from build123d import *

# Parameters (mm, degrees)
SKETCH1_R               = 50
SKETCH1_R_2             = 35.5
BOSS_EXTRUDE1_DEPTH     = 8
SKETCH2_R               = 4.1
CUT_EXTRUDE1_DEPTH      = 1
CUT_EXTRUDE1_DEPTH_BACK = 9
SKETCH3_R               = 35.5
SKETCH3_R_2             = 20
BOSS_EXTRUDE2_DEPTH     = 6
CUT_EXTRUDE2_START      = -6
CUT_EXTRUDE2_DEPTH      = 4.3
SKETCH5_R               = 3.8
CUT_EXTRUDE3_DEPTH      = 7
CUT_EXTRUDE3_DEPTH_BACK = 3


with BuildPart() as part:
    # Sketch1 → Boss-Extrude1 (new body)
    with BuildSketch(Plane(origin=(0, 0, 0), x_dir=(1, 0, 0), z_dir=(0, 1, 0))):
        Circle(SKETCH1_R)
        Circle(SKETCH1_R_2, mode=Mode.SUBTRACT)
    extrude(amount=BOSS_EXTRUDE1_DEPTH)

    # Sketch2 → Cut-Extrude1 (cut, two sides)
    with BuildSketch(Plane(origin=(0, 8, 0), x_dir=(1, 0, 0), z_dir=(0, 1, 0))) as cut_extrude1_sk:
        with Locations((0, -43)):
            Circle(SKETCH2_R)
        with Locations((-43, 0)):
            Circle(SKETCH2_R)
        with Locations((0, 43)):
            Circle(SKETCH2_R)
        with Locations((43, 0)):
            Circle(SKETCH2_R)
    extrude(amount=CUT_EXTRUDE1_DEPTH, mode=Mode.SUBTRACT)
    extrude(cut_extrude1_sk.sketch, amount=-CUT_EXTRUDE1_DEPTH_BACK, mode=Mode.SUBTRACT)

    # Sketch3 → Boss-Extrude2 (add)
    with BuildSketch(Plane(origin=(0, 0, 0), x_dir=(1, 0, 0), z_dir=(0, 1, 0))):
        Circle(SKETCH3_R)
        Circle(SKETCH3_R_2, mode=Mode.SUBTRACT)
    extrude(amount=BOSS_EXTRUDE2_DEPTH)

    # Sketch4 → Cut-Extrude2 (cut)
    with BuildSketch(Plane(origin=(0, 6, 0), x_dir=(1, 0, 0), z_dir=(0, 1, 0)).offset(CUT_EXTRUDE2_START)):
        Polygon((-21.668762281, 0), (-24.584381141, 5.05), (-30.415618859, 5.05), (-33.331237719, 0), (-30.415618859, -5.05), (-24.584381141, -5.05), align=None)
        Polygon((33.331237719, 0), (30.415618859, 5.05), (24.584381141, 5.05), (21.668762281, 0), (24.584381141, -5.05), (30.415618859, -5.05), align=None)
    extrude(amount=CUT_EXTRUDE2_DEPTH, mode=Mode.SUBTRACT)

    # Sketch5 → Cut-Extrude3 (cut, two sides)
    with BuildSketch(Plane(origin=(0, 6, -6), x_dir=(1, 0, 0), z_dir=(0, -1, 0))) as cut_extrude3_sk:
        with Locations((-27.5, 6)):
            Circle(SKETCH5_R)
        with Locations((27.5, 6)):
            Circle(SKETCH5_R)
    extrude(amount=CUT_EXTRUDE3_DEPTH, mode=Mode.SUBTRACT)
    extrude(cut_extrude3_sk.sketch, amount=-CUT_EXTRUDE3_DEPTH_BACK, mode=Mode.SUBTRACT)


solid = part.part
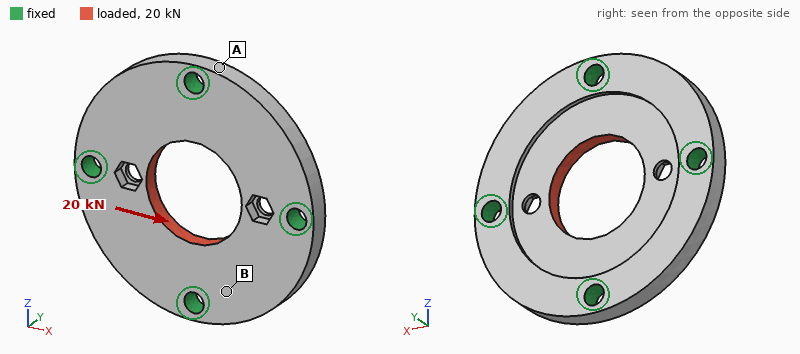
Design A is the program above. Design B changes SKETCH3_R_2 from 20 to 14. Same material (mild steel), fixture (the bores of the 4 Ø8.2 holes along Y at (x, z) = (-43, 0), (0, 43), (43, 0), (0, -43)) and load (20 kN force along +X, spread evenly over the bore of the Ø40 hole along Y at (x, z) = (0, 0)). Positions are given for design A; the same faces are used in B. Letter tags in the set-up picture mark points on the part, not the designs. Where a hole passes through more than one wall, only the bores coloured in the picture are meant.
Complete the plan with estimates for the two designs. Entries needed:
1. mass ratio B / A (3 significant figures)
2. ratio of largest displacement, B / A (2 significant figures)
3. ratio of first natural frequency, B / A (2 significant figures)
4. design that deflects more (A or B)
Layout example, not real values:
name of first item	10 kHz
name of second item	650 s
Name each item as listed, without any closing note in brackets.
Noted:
mass ratio B / A	1.09
ratio of largest displacement, B / A	0.86
ratio of first natural frequency, B / A	0.92
design that deflects more	A
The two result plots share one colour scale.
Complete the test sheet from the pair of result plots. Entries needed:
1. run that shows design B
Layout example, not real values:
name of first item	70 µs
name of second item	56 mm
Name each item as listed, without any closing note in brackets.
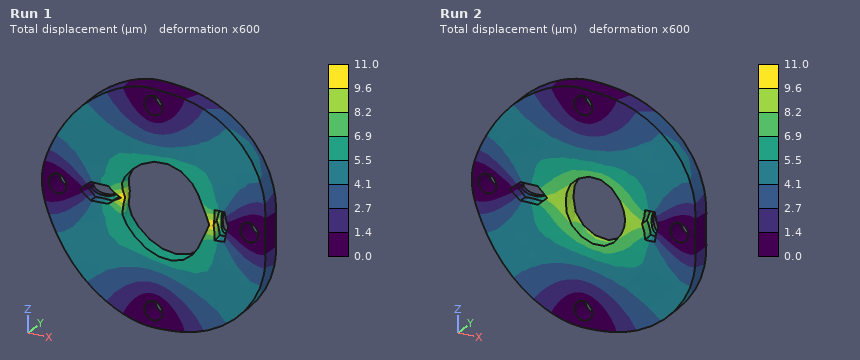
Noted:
run that shows design B	Run 2
